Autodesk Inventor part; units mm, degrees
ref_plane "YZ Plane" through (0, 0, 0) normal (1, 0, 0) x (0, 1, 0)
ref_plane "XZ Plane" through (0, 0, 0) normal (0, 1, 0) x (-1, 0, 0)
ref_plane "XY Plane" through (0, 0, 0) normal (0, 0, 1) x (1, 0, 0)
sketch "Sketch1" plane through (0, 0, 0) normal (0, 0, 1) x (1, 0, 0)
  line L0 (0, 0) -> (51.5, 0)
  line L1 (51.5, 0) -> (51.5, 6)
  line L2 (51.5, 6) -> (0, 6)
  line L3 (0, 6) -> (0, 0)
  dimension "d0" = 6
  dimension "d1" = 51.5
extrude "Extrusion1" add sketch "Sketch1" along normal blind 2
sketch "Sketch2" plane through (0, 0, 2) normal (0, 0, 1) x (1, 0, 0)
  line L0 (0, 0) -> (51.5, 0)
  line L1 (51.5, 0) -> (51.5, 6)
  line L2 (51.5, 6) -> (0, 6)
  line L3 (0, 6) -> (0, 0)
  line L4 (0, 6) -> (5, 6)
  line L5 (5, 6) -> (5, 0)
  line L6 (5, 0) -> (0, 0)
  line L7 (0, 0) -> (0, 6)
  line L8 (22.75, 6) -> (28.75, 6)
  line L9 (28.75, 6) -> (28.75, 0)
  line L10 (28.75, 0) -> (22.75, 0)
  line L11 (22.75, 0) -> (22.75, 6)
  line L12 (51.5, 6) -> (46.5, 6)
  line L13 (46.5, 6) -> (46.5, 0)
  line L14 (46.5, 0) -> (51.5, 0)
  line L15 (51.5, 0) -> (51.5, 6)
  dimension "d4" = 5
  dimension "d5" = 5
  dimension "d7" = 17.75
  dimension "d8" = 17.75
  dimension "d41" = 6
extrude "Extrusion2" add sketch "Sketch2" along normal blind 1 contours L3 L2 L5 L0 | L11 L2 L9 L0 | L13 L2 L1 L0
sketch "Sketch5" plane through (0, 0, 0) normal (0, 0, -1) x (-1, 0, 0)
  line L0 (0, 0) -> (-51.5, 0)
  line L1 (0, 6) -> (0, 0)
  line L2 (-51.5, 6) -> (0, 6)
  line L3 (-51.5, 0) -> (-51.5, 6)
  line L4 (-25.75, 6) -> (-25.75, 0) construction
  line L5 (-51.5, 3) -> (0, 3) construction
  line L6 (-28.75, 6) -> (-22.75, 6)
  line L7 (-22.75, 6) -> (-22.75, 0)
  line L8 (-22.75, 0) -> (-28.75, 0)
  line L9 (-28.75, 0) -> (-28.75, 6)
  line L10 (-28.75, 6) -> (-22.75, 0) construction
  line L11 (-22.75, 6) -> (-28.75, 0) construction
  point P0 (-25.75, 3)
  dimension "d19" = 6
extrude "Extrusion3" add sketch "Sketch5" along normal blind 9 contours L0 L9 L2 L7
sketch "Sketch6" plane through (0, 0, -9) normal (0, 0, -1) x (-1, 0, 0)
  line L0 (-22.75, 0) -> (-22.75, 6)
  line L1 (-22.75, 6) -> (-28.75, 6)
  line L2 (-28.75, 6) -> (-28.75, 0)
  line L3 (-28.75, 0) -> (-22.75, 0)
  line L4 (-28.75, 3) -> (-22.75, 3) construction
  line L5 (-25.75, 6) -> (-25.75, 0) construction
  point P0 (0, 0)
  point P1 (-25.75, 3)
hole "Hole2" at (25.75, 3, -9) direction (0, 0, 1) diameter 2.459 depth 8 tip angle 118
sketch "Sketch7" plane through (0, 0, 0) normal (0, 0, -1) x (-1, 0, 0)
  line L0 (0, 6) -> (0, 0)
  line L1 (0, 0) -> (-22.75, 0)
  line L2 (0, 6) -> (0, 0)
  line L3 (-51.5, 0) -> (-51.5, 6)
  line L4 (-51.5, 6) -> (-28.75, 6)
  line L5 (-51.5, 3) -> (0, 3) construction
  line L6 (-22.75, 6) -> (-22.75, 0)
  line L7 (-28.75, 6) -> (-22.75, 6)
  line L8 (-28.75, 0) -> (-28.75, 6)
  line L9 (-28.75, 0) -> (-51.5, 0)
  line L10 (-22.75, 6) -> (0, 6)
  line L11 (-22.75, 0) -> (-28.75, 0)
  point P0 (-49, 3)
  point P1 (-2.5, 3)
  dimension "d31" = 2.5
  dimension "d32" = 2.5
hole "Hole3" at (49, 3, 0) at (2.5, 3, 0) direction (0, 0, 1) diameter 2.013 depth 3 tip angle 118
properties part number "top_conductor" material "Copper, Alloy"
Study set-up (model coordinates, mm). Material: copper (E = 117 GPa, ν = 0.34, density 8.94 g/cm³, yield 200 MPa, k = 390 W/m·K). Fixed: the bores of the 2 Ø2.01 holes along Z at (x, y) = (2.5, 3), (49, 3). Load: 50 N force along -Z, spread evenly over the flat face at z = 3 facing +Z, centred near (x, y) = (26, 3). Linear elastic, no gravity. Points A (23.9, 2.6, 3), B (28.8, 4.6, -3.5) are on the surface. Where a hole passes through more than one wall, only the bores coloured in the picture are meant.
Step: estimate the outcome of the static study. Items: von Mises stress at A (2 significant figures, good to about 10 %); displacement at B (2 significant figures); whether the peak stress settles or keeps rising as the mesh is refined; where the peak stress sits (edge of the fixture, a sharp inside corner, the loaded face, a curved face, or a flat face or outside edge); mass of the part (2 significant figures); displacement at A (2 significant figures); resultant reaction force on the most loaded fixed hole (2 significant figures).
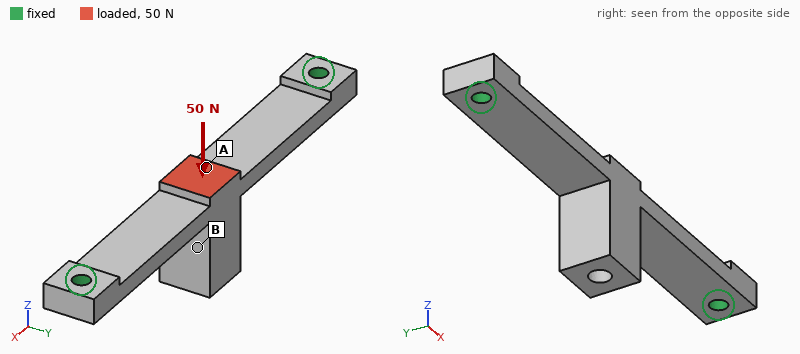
9.2 MPa
34 µm
keeps rising
edge of the fixture
8.8 g
34 µm
27 N
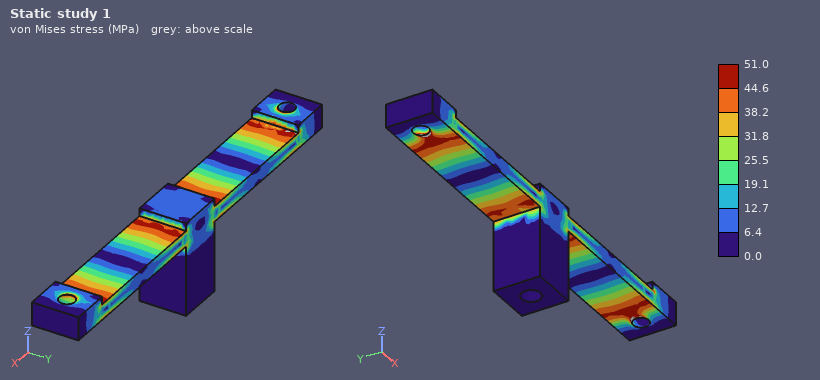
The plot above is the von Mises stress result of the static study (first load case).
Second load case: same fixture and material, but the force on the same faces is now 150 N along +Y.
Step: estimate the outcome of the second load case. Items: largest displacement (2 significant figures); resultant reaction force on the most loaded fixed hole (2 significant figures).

36 µm
75 N
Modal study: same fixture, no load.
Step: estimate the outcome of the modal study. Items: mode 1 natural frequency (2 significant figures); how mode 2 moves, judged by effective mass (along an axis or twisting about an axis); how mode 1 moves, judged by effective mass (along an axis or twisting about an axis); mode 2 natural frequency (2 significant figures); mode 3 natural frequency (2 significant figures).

2700 Hz
along Y
along Z
3500 Hz
6500 Hz
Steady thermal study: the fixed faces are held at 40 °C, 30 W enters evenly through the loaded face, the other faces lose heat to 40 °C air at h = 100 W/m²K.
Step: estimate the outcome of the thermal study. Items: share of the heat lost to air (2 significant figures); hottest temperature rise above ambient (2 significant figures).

13 %
62 K
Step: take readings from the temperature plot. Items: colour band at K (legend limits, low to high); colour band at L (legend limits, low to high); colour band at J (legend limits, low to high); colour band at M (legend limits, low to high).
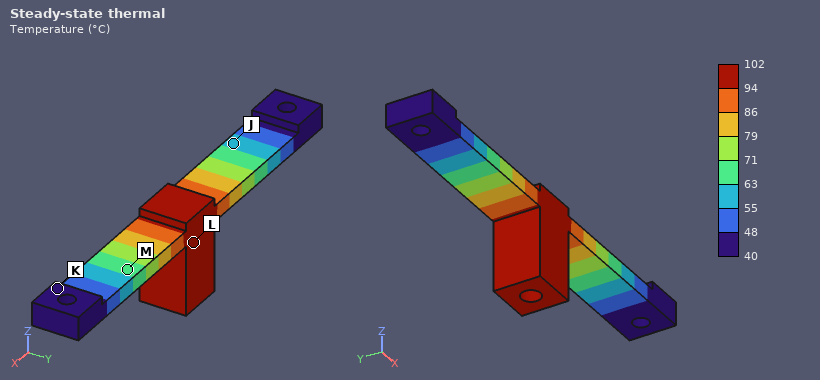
40 to 48 °C
94 to 102 °C
55 to 63 °C
63 to 71 °C
